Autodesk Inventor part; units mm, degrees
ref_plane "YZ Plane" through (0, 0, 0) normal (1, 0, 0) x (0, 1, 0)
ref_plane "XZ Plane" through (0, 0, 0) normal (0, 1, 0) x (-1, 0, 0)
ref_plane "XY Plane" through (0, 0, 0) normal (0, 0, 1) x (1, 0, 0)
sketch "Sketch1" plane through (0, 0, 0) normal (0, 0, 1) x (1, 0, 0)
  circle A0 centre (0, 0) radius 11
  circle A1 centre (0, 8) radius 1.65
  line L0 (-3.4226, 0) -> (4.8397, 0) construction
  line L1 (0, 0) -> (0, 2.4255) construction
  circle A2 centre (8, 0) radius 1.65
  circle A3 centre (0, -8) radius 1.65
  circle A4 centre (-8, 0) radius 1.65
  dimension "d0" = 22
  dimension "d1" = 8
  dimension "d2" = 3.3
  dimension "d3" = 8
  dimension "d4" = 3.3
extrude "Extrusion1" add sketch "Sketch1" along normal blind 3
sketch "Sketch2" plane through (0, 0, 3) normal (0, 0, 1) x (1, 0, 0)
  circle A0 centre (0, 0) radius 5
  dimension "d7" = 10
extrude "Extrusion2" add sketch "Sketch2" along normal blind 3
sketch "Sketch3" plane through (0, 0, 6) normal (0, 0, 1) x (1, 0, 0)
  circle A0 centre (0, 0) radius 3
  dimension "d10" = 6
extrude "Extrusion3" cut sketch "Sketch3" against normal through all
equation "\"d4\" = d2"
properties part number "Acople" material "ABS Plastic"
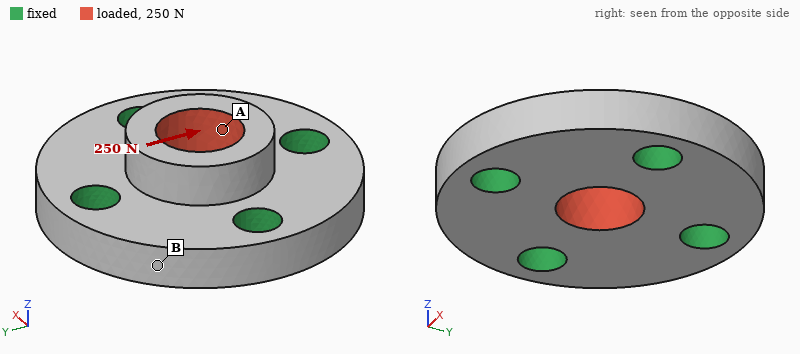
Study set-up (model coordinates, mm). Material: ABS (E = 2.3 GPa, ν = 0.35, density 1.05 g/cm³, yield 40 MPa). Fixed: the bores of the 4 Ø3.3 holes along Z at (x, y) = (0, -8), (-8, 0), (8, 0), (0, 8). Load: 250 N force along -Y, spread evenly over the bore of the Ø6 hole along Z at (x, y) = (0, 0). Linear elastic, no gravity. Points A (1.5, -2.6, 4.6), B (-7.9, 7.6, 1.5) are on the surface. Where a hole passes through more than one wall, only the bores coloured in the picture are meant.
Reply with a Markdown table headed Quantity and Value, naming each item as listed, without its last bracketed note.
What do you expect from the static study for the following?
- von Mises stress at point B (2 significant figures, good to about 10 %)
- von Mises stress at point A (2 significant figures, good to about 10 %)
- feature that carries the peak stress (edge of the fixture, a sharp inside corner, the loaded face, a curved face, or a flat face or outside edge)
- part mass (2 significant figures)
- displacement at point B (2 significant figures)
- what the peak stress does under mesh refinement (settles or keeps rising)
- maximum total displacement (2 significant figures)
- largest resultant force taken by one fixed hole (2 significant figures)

| Quantity | Value |
|---|---|
| von Mises stress at point B | 1.2 MPa |
| von Mises stress at point A | 4.5 MPa |
| feature that carries the peak stress | a sharp inside corner |
| part mass | 1.2 g |
| displacement at point B | 3.8 µm |
| what the peak stress does under mesh refinement | keeps rising |
| maximum total displacement | 24 µm |
| largest resultant force taken by one fixed hole | 84 N |
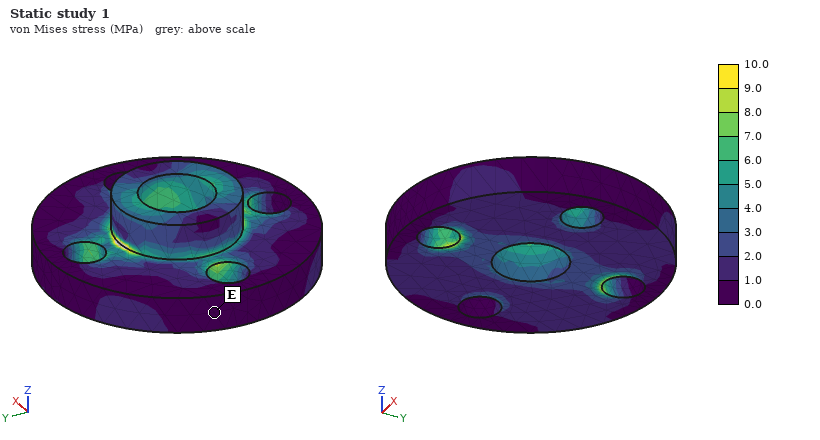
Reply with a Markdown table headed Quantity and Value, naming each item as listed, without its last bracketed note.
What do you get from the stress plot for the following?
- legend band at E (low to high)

| Quantity | Value |
|---|---|
| legend band at E | 0.0 to 1.0 MPa |
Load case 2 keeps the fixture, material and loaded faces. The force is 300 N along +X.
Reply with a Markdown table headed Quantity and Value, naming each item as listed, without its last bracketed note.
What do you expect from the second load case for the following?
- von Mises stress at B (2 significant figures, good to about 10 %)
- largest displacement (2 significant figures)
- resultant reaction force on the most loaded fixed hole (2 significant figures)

| Quantity | Value |
|---|---|
| von Mises stress at B | 1.5 MPa |
| largest displacement | 29 µm |
| resultant reaction force on the most loaded fixed hole | 100 N |
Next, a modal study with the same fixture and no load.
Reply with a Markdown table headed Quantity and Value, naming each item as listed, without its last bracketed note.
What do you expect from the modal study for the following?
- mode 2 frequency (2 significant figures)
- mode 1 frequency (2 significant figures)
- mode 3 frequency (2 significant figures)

| Quantity | Value |
|---|---|
| mode 2 frequency | 25 kHz |
| mode 1 frequency | 24 kHz |
| mode 3 frequency | 25 kHz |
